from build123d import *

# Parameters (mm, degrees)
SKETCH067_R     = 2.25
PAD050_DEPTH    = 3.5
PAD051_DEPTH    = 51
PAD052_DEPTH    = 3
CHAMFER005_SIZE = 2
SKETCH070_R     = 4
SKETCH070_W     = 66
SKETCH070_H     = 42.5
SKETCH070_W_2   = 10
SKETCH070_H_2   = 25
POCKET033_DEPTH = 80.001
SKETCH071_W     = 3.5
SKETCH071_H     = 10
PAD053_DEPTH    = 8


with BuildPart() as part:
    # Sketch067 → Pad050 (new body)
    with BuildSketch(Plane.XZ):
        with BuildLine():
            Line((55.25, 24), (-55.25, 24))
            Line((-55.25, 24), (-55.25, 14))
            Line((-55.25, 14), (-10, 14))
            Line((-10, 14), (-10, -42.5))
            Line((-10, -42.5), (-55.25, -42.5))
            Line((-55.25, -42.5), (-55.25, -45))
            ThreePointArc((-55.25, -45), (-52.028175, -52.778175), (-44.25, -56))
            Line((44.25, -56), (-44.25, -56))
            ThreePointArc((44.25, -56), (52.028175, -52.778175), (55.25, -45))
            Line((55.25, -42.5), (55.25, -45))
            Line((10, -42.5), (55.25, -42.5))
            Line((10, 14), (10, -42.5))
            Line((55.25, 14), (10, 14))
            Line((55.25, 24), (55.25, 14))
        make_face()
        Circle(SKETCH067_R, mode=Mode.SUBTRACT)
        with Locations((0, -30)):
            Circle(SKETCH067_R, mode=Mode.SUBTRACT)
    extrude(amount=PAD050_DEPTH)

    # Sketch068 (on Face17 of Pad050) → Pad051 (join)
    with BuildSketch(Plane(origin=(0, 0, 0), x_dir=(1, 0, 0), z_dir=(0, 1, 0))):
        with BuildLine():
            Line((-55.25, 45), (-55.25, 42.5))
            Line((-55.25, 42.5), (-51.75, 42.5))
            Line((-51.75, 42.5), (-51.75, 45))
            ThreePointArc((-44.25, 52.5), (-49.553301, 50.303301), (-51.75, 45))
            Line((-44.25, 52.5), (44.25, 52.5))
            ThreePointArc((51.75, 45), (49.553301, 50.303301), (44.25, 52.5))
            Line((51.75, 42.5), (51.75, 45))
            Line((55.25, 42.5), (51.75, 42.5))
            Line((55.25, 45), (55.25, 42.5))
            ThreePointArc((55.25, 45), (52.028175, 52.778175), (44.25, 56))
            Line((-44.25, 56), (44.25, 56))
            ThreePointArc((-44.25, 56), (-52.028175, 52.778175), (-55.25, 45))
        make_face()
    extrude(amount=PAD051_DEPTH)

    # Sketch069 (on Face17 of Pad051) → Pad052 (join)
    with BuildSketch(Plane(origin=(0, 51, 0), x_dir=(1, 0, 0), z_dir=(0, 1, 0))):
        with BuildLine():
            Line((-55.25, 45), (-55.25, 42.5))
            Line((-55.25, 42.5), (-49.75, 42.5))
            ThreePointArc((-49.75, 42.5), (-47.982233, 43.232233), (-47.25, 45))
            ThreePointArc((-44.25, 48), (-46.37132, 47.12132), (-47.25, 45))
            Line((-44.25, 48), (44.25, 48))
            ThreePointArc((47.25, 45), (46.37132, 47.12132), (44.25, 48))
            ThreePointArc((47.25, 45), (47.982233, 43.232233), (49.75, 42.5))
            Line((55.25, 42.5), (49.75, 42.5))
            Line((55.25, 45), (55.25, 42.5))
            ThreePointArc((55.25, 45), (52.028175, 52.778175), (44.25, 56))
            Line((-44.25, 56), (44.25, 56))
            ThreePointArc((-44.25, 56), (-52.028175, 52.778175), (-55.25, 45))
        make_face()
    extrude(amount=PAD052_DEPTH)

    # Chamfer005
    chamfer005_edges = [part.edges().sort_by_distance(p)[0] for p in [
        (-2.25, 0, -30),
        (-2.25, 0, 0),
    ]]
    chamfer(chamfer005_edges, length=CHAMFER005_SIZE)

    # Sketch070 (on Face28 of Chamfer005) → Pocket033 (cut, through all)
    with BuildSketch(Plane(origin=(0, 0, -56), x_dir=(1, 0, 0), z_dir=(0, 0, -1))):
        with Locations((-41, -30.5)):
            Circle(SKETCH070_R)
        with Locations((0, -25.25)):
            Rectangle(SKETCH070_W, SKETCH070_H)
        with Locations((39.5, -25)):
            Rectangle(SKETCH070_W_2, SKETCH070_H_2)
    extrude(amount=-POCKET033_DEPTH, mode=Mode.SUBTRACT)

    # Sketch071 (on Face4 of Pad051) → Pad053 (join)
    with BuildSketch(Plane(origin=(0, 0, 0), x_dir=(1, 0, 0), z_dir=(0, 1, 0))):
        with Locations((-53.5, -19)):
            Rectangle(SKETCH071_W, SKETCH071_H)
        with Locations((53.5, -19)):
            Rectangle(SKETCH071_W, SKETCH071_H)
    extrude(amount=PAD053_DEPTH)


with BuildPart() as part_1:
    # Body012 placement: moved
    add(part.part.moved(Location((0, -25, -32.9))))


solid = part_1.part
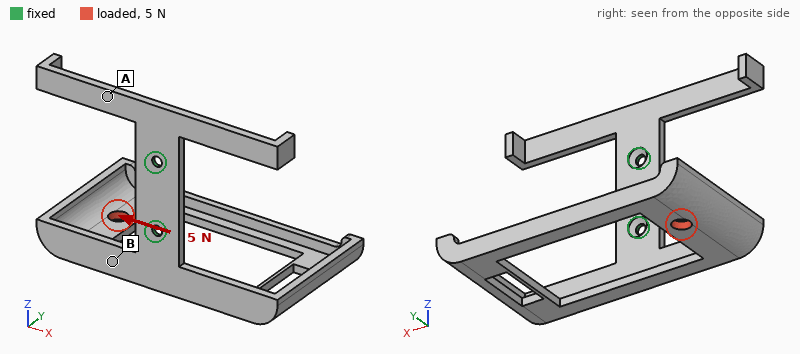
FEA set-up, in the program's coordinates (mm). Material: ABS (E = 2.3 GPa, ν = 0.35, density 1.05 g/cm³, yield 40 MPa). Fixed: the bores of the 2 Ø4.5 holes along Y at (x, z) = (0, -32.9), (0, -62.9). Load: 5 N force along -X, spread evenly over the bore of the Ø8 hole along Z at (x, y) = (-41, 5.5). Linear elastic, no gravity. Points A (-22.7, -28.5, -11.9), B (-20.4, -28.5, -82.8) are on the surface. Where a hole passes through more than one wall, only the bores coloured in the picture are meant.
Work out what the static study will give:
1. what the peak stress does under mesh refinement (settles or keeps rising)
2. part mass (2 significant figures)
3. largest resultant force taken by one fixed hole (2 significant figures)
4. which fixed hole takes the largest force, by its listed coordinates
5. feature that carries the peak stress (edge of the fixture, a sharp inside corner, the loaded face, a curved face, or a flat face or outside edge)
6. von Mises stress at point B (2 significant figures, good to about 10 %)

keeps rising
28 g
7.2 N
(0, -62.9)
edge of the fixture
0.89 MPa
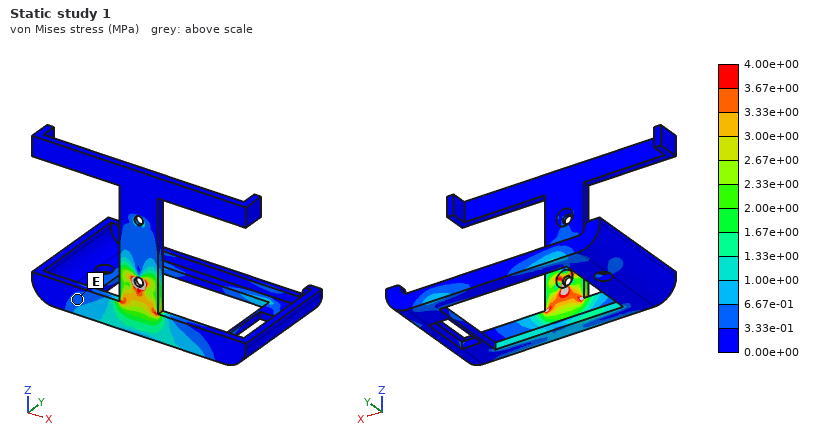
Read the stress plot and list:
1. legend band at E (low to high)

3.33e-01 to 6.67e-01 MPa
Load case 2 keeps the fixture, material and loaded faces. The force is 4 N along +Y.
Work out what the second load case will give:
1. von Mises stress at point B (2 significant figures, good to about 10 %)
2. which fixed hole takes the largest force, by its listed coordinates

0.65 MPa
(0, -62.9)
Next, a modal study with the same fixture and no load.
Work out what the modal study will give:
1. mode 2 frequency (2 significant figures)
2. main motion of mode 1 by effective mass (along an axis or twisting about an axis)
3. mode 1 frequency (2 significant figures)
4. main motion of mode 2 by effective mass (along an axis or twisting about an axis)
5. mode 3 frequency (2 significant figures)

73 Hz
along X
67 Hz
along Z
170 Hz
